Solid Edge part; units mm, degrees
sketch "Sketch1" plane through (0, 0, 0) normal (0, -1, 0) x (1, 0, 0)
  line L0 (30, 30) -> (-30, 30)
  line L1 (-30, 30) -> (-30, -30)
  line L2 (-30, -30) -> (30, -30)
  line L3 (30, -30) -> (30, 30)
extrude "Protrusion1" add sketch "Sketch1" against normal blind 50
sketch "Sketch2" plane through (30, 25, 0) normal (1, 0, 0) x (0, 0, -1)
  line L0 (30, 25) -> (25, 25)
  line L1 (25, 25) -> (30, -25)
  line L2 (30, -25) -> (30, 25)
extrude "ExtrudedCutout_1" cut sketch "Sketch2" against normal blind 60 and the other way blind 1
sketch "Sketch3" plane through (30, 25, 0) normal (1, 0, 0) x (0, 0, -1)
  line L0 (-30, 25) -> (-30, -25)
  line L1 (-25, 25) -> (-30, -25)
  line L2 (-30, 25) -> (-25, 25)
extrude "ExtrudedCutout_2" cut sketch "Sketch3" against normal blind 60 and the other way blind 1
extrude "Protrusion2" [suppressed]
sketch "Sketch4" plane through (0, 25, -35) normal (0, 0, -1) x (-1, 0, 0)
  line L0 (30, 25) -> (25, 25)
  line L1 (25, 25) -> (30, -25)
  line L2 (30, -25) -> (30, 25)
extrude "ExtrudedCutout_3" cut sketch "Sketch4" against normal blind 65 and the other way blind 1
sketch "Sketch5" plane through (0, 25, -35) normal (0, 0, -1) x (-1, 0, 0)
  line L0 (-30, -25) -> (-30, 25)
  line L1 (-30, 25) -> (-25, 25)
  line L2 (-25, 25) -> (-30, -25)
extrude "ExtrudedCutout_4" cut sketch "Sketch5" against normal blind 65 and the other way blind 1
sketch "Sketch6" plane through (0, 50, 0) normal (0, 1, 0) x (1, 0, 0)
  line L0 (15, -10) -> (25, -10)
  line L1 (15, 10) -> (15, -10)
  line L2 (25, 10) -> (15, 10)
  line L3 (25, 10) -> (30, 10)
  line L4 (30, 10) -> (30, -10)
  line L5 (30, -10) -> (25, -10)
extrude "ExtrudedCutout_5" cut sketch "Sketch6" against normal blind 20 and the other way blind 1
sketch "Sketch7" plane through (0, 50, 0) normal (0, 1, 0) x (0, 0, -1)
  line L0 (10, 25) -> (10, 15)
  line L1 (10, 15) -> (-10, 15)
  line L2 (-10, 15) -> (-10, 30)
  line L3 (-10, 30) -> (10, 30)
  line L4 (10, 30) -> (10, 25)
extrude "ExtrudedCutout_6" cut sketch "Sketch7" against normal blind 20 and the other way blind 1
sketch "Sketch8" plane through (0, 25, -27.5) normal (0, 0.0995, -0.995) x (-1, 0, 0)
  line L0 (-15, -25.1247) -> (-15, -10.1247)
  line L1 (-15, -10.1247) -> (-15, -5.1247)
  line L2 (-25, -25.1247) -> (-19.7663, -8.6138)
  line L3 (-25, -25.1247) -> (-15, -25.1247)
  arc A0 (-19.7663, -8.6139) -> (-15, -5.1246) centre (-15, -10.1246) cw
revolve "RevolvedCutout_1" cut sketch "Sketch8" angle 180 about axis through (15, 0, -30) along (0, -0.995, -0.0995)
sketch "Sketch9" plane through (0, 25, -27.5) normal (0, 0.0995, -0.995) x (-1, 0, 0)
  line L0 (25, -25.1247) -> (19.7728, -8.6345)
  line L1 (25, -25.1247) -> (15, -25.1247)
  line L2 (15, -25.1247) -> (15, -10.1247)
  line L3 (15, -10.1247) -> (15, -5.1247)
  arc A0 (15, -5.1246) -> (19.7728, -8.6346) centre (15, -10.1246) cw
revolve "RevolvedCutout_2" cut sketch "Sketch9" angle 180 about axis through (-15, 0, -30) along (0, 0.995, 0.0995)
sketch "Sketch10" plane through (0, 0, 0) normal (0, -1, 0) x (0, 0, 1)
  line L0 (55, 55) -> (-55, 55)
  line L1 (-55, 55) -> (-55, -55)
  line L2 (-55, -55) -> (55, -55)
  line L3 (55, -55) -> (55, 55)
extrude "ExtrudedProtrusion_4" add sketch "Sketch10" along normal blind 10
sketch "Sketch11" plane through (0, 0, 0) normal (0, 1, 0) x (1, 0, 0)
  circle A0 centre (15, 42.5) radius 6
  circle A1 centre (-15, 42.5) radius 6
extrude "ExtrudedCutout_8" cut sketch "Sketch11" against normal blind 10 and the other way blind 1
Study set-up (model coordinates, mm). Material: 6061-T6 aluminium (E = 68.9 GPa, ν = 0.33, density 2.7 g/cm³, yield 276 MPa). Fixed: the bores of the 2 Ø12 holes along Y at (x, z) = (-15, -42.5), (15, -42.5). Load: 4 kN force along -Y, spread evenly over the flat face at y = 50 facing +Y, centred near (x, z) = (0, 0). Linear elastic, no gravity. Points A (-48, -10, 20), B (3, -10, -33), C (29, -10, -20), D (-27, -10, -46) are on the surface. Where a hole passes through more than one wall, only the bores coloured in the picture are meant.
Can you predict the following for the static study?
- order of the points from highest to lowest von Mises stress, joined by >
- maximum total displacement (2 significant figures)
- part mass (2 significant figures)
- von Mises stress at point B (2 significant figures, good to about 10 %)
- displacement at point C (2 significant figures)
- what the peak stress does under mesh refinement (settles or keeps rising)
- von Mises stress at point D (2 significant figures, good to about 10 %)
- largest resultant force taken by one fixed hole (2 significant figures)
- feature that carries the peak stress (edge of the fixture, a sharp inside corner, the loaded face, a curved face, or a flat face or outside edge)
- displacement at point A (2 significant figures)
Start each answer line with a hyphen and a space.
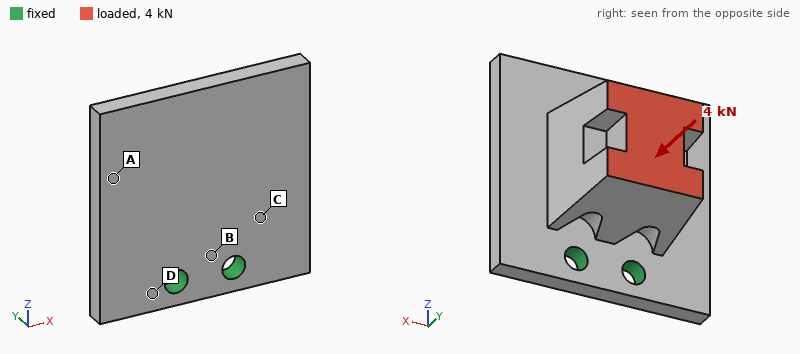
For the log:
- B > D > C > A
- 0.40 mm
- 700 g
- 73 MPa
- 0.065 mm
- keeps rising
- 39 MPa
- 2.0 kN
- edge of the fixture
- 0.24 mm
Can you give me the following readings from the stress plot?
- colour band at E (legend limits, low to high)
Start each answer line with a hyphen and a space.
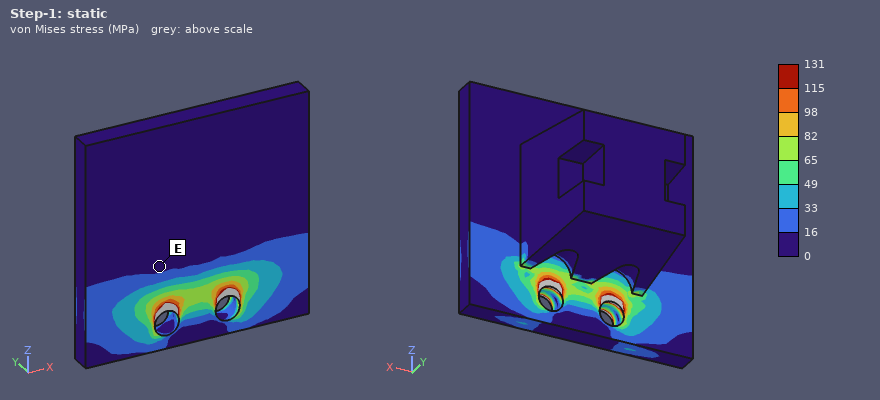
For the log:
- 0 to 16 MPa
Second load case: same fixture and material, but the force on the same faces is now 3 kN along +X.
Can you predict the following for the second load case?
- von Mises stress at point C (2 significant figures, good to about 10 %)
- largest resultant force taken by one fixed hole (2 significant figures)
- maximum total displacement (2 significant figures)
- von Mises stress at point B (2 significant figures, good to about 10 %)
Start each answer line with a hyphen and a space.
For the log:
- 14 MPa
- 5.0 kN
- 86 µm
- 13 MPa
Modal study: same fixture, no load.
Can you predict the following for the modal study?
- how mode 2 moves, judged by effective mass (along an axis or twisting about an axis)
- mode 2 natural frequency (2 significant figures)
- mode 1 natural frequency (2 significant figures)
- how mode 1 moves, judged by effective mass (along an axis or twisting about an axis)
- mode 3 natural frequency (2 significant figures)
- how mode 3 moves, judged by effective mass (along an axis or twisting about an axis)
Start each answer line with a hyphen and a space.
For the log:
- along X
- 2000 Hz
- 680 Hz
- along Y
- 2700 Hz
- along X
